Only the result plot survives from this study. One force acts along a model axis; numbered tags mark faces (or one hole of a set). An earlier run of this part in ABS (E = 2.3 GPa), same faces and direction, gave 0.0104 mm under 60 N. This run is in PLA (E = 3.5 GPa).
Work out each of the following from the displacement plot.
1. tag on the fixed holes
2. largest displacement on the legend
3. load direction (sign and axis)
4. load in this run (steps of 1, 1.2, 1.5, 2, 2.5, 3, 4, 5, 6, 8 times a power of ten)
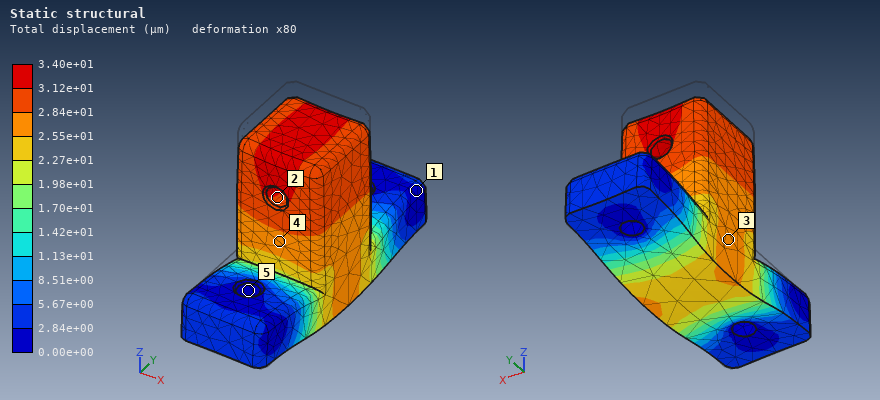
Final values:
5
3.40e+01 µm
-Z
300 N
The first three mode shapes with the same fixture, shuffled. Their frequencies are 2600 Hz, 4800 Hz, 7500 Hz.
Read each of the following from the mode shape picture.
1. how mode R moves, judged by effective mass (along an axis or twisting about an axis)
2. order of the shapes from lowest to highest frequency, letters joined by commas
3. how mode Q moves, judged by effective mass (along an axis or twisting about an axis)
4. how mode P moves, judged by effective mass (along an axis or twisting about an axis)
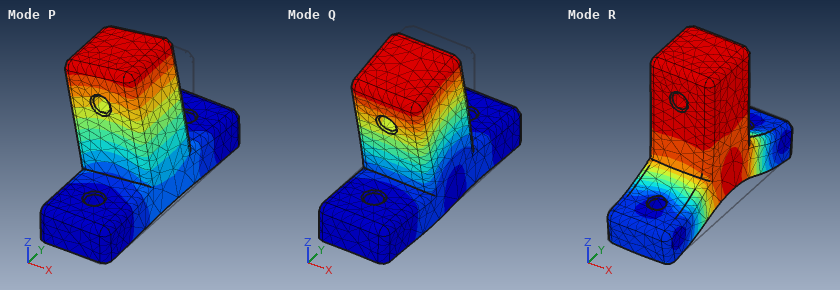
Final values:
along Z
P, Q, R
along Y
along X
